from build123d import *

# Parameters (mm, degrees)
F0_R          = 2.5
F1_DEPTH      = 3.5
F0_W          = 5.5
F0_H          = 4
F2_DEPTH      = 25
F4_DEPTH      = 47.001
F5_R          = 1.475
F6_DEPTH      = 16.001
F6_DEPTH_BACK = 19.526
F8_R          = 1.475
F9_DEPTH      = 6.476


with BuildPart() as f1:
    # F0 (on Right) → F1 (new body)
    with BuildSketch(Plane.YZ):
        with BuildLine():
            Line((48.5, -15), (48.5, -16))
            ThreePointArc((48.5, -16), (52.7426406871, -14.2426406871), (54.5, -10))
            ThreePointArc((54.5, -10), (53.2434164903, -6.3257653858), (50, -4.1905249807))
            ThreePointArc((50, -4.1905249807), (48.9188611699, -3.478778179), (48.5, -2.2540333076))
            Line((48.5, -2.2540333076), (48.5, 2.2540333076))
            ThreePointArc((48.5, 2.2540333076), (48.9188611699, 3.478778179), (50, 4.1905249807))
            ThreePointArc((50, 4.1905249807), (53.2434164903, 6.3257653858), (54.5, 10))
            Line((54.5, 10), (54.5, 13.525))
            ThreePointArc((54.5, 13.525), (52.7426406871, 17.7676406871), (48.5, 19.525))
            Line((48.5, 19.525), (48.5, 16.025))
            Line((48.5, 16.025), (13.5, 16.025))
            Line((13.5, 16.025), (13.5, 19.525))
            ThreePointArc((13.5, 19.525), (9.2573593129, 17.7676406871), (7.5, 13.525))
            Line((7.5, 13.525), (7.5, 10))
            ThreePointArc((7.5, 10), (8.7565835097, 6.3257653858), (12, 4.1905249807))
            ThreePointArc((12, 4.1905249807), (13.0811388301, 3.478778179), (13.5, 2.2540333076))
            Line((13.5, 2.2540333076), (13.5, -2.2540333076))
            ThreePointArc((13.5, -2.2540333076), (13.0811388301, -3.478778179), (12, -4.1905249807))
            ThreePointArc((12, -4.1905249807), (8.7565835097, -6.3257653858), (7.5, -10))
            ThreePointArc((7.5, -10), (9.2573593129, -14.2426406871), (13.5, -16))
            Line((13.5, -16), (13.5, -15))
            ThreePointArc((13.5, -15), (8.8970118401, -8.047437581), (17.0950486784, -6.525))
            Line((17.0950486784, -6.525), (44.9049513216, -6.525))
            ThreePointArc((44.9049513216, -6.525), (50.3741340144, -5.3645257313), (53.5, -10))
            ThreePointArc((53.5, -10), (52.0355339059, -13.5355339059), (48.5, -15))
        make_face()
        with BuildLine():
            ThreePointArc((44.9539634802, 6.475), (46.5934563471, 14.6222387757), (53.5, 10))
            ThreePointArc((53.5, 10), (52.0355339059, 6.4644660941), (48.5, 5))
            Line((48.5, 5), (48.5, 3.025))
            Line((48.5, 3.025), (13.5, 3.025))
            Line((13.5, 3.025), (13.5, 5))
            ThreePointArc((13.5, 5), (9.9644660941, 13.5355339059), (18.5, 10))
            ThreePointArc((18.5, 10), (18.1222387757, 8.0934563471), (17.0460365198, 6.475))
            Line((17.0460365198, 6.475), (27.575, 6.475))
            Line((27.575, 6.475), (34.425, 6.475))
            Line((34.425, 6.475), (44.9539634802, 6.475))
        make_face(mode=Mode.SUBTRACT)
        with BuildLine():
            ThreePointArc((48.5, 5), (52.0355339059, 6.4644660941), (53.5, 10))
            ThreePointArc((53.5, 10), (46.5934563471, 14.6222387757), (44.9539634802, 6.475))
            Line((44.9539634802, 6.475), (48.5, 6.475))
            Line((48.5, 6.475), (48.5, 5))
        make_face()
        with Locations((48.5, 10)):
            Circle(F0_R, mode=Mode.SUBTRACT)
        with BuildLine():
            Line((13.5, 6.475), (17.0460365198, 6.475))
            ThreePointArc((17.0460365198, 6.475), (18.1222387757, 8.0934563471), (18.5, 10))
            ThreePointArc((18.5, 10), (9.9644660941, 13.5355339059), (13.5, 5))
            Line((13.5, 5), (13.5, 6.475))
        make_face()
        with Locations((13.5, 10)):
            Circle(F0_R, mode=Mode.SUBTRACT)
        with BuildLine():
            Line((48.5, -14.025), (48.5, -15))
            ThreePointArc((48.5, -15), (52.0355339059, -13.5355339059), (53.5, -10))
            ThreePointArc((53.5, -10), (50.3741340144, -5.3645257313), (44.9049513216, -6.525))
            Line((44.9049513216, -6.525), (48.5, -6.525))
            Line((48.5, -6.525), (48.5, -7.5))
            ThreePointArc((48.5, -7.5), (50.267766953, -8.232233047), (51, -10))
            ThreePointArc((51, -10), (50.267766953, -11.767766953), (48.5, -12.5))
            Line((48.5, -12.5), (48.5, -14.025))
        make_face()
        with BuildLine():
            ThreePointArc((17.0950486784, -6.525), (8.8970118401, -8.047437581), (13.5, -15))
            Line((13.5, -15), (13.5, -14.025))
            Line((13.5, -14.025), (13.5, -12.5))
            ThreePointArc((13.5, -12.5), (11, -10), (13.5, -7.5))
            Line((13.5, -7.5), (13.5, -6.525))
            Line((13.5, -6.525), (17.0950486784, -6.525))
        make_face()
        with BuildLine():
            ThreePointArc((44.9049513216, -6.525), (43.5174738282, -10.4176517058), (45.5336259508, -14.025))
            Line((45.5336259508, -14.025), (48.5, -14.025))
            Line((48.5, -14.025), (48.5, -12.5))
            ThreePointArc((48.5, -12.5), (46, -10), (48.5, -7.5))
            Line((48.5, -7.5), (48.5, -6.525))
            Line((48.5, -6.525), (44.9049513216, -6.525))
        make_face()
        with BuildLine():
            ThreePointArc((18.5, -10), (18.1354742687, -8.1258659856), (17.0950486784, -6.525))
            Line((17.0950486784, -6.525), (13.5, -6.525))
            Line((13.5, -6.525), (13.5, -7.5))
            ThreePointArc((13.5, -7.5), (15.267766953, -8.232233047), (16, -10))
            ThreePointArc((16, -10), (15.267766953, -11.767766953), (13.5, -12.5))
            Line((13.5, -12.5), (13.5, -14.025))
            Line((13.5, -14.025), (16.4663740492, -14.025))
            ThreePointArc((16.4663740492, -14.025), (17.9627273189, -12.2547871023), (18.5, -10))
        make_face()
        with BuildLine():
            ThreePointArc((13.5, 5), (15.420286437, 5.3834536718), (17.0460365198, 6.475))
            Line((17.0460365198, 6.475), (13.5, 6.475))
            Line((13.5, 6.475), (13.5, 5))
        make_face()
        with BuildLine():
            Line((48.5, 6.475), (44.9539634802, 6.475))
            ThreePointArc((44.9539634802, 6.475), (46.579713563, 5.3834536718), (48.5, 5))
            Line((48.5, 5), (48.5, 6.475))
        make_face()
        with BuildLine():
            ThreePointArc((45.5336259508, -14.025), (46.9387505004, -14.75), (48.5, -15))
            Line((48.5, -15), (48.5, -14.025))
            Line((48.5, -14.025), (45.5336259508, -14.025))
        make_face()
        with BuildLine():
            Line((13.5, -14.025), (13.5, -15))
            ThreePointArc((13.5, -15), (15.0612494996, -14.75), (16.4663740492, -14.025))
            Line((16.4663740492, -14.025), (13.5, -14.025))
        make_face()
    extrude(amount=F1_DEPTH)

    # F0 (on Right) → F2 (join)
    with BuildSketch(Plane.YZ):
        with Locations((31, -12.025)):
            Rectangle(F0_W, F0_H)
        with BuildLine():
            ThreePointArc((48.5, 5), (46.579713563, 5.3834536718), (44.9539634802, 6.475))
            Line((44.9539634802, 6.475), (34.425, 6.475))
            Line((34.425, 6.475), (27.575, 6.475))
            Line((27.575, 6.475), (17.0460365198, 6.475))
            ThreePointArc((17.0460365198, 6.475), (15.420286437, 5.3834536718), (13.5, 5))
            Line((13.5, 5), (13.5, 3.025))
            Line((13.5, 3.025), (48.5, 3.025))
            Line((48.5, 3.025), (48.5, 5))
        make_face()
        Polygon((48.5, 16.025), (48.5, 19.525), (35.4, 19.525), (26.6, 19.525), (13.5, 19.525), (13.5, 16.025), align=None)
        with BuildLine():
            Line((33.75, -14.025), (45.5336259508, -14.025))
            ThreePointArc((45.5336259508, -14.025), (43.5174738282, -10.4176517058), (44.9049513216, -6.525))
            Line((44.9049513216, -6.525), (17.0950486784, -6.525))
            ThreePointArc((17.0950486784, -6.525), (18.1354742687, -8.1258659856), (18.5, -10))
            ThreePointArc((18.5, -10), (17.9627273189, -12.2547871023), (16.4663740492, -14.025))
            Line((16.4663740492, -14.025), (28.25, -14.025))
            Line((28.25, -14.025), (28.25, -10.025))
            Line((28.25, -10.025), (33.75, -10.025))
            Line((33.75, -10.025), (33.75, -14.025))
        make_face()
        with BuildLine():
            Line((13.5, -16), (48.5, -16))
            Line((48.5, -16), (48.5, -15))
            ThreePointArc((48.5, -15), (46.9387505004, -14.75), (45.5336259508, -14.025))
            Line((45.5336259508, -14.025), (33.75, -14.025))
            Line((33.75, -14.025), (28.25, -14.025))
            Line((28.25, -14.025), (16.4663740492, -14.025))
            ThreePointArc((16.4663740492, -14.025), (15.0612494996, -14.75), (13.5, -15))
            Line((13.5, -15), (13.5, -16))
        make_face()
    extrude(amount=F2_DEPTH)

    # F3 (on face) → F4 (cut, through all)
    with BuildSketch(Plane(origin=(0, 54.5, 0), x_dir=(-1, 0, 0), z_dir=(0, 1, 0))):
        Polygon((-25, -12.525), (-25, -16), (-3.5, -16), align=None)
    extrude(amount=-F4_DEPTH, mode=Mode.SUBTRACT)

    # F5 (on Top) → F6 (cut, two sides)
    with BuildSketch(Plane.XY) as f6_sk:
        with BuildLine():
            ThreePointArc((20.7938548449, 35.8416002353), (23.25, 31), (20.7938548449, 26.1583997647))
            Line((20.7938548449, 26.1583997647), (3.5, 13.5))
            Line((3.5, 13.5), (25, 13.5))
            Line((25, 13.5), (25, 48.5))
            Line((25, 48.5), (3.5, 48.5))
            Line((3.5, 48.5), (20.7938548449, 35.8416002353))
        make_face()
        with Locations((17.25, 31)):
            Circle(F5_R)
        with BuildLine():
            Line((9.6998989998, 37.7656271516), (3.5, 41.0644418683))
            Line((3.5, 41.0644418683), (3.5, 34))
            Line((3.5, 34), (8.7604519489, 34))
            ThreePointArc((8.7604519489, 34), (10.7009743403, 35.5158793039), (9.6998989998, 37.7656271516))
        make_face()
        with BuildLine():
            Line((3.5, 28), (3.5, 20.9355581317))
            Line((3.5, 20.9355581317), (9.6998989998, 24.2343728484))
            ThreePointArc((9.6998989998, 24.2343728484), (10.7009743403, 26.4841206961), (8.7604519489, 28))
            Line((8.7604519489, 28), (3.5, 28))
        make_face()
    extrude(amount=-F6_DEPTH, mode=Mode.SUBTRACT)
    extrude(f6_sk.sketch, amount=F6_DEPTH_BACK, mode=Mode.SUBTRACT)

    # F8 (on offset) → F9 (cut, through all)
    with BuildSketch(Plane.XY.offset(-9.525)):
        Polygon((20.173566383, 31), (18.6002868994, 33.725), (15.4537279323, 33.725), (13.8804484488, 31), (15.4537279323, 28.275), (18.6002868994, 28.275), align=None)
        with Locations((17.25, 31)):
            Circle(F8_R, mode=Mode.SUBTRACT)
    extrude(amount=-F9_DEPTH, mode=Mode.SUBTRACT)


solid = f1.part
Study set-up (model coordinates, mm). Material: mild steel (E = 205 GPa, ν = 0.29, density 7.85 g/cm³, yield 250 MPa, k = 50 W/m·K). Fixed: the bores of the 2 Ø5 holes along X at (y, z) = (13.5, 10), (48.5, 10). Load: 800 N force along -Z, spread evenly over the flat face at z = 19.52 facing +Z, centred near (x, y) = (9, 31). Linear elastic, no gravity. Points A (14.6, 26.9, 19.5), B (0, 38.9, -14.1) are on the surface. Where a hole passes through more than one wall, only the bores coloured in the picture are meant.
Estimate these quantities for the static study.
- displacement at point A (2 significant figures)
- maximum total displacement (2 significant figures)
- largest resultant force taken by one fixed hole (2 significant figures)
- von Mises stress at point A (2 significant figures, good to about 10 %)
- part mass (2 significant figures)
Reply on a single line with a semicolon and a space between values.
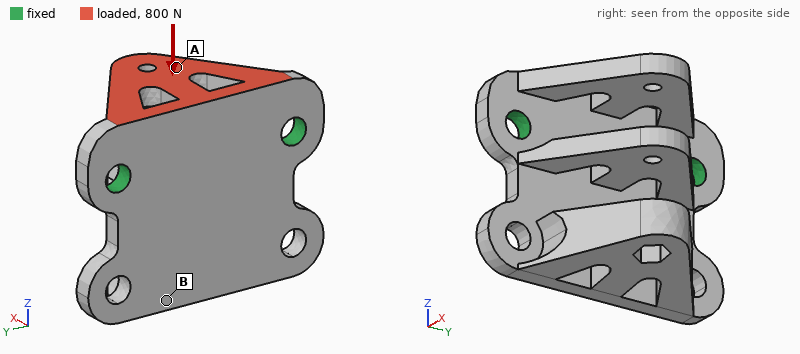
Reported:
43 µm; 78 µm; 400 N; 25 MPa; 75 g
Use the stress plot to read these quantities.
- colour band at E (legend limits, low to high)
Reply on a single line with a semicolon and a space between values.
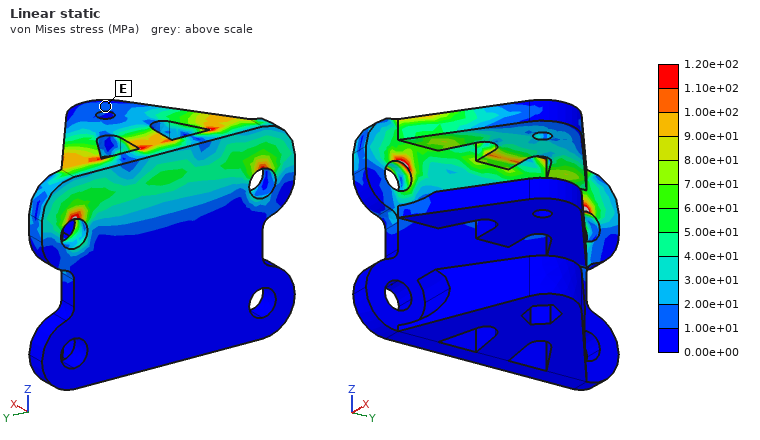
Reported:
1.00e+01 to 2.00e+01 MPa
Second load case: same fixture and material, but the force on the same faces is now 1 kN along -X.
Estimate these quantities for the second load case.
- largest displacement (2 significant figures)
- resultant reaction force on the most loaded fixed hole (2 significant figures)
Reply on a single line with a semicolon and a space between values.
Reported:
47 µm; 530 N
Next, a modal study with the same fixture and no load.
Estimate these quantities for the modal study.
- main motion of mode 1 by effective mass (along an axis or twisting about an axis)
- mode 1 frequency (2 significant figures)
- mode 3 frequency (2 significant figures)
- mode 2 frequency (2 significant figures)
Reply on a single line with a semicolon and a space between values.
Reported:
along X; 2300 Hz; 6000 Hz; 5700 Hz
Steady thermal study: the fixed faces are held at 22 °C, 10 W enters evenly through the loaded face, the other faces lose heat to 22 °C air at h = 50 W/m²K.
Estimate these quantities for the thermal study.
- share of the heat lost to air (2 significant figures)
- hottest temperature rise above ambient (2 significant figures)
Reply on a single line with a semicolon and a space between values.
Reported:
20 %; 35 K
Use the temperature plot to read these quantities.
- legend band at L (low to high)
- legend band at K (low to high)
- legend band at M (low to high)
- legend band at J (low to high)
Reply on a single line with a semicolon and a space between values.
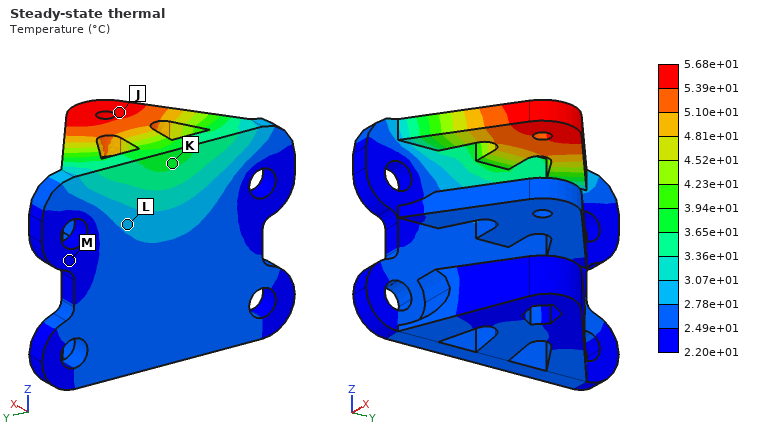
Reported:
2.78e+01 to 3.07e+01 °C; 3.65e+01 to 3.94e+01 °C; 2.20e+01 to 2.49e+01 °C; 5.39e+01 to 5.68e+01 °C
